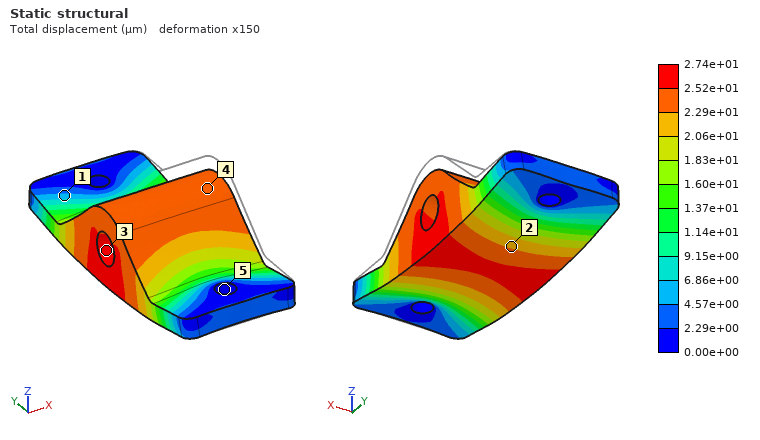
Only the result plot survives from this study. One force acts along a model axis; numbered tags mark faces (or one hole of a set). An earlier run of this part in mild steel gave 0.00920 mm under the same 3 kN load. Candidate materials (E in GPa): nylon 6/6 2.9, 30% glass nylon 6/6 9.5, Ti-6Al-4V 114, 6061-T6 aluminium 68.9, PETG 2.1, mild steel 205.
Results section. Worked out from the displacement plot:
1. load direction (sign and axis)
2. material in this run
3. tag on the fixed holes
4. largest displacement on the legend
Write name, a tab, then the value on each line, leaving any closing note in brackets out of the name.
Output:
load direction	-Z
material in this run	6061-T6 aluminium
tag on the fixed holes	5
largest displacement on the legend	2.74e+01 µm
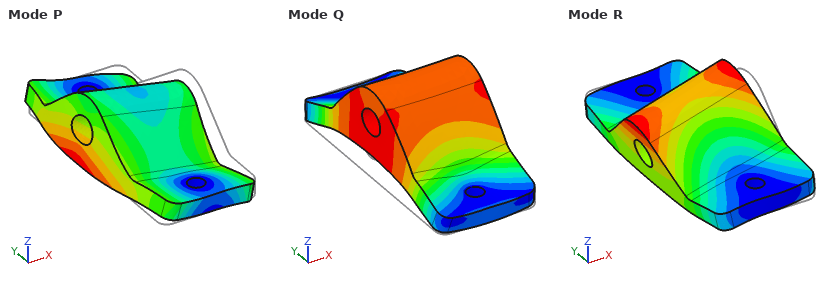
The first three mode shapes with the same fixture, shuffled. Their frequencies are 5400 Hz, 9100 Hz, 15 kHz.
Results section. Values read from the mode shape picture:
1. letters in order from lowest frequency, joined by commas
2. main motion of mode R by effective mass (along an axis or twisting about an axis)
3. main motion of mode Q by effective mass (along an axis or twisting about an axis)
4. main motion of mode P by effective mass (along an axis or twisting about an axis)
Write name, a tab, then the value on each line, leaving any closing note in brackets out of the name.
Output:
letters in order from lowest frequency, joined by commas	R, Q, P
main motion of mode R by effective mass	along X
main motion of mode Q by effective mass	along Z
main motion of mode P by effective mass	along X
